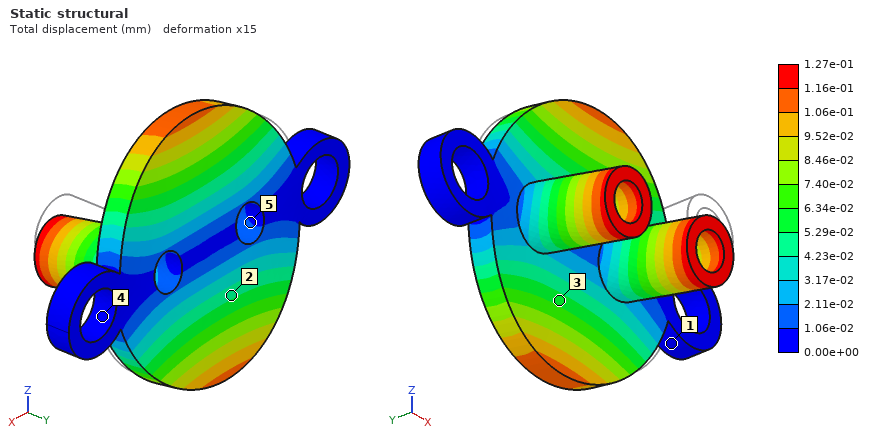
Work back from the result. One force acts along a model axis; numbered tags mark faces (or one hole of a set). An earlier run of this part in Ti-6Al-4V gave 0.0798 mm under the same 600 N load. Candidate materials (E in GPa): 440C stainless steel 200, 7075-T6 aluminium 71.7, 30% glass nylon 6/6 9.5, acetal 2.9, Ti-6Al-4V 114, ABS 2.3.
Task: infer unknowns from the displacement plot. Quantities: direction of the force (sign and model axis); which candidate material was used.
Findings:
-Z
7075-T6 aluminium
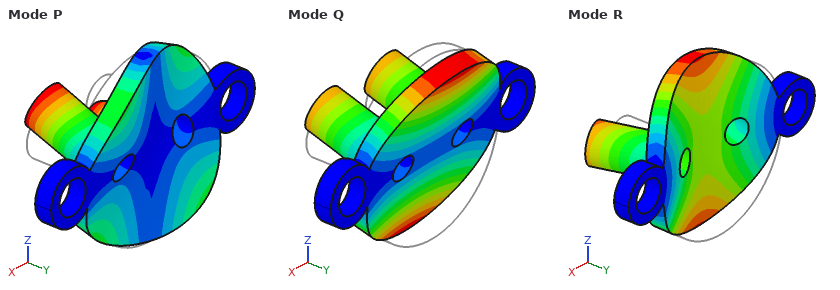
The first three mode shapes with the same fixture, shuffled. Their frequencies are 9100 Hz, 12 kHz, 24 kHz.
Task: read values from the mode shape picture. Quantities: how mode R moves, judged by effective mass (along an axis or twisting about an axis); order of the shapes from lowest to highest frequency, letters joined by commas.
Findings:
along Y
Q, R, P
